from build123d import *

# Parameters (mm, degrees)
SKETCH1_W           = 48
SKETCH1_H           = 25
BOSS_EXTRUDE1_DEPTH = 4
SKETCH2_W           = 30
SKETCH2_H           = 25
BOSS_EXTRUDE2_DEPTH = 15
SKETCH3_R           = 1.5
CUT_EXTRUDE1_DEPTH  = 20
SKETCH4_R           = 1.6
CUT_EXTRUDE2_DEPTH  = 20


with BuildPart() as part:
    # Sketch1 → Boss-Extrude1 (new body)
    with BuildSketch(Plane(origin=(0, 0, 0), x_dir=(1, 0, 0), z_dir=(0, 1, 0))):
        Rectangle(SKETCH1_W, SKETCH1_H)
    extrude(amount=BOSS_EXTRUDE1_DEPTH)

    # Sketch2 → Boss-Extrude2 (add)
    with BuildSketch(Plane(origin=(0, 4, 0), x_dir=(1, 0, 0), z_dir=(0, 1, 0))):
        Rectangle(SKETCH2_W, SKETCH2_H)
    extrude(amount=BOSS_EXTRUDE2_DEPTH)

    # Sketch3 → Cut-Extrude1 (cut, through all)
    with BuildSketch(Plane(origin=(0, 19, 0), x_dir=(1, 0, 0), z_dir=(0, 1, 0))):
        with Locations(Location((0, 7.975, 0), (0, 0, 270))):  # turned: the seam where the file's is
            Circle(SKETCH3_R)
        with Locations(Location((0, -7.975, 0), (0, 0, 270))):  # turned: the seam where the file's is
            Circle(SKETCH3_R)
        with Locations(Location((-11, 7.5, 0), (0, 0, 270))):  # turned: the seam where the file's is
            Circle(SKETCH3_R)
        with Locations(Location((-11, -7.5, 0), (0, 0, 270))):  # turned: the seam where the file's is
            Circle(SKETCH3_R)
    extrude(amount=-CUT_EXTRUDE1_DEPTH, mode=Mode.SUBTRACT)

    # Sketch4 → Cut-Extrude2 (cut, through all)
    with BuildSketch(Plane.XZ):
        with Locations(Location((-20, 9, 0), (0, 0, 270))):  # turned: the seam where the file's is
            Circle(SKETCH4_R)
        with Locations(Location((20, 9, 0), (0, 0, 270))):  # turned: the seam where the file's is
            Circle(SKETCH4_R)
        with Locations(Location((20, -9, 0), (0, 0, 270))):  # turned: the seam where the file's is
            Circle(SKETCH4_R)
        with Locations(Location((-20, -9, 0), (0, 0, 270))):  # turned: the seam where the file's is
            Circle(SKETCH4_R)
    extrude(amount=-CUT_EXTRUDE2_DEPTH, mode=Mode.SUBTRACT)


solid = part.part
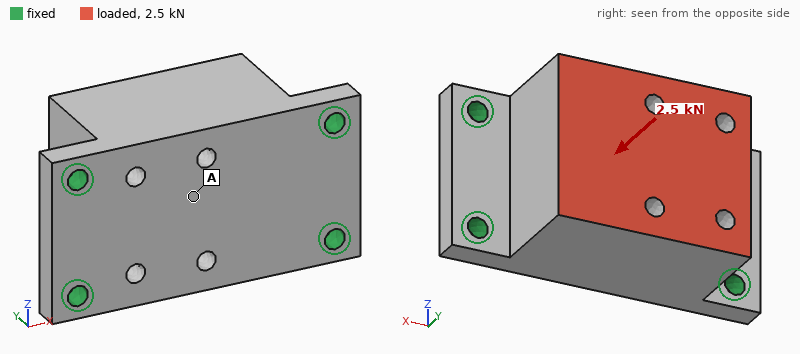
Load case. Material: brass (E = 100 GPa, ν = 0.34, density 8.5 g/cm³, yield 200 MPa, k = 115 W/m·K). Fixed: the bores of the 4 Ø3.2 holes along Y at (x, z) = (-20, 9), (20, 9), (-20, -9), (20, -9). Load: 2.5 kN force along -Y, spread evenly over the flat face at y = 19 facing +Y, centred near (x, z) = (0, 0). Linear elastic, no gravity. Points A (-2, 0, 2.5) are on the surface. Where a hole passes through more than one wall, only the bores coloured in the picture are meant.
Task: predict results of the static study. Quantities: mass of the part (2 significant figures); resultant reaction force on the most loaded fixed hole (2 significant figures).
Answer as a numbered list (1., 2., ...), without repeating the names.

1. 130 g
2. 710 N
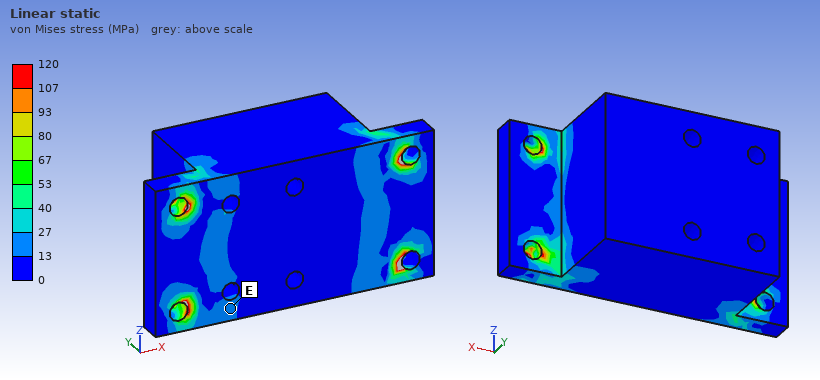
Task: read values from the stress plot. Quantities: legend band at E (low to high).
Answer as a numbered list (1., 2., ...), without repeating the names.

1. 13 to 27 MPa
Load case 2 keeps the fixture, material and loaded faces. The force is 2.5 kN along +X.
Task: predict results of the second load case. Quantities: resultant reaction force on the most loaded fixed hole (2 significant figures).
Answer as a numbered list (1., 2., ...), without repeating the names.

1. 900 N
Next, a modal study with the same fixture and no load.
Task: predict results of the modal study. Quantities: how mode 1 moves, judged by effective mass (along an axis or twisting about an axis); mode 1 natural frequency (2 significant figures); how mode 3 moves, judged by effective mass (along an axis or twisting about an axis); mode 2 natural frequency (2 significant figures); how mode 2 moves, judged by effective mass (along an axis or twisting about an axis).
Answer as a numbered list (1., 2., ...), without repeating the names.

1. along Z
2. 6600 Hz
3. along X
4. 9200 Hz
5. along Y
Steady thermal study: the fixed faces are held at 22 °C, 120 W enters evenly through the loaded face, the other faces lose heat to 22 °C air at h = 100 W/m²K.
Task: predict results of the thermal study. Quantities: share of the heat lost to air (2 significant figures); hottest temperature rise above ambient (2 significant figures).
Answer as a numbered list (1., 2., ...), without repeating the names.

1. 14 %
2. 63 K
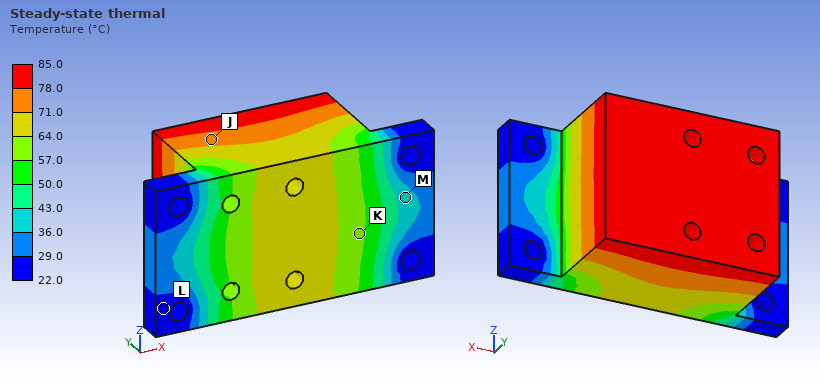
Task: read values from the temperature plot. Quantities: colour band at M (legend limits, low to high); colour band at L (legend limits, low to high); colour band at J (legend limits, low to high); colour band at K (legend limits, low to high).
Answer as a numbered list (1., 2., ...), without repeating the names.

1. 36.0 to 43.0 °C
2. 22.0 to 29.0 °C
3. 71.0 to 78.0 °C
4. 57.0 to 64.0 °C
